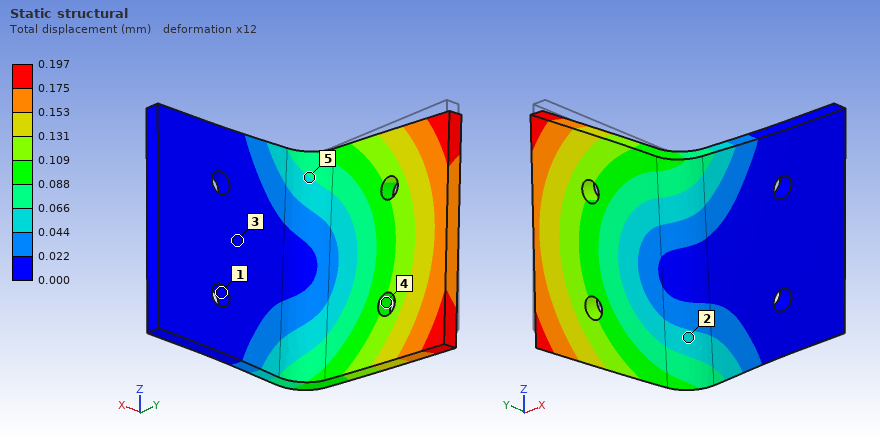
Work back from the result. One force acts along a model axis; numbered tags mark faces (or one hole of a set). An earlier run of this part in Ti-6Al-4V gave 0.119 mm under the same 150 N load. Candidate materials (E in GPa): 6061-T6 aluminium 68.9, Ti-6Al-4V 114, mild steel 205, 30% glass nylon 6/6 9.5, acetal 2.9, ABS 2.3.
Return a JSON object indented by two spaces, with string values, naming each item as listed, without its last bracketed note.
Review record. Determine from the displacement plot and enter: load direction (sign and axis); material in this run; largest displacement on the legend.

{
  "load direction": "-Z",
  "material in this run": "6061-T6 aluminium",
  "largest displacement on the legend": "0.197 mm"
}
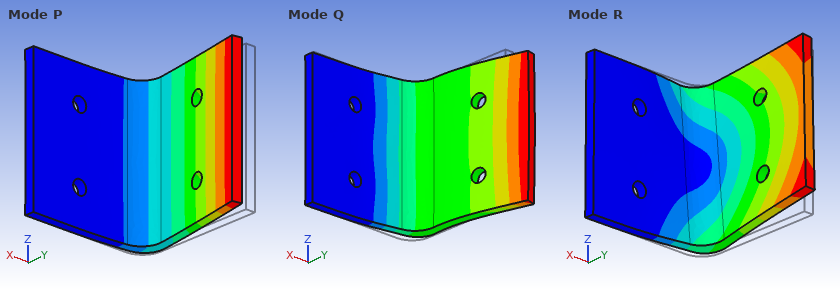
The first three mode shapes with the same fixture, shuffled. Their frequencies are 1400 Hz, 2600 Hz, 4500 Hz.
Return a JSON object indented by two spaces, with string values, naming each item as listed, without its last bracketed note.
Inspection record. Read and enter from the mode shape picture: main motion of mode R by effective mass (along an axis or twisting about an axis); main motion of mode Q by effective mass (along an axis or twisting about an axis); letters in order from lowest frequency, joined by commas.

{
  "main motion of mode R by effective mass": "along Z",
  "main motion of mode Q by effective mass": "along Y",
  "letters in order from lowest frequency, joined by commas": "P, R, Q"
}
